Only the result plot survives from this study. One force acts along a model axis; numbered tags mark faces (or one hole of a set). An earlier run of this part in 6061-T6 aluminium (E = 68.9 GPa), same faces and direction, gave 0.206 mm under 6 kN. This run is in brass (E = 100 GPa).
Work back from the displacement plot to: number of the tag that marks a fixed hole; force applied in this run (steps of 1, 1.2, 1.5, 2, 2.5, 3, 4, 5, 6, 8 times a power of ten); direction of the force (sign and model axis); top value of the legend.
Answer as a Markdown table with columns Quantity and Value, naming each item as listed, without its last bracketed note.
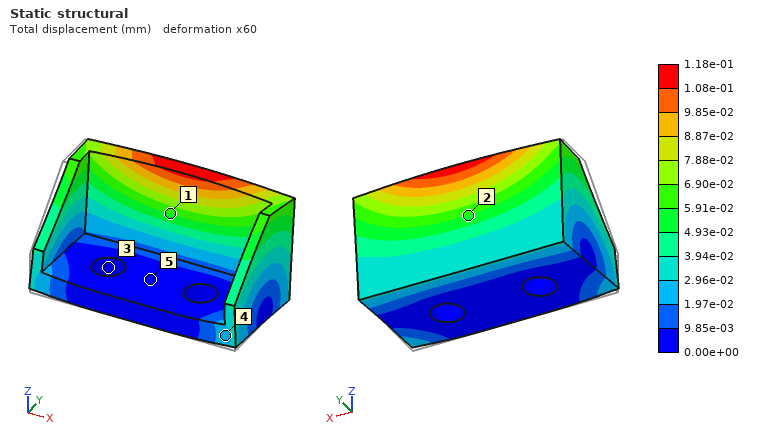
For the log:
| Quantity | Value |
|---|---|
| number of the tag that marks a fixed hole | 3 |
| force applied in this run | 5 kN |
| direction of the force | +Y |
| top value of the legend | 1.18e-01 mm |
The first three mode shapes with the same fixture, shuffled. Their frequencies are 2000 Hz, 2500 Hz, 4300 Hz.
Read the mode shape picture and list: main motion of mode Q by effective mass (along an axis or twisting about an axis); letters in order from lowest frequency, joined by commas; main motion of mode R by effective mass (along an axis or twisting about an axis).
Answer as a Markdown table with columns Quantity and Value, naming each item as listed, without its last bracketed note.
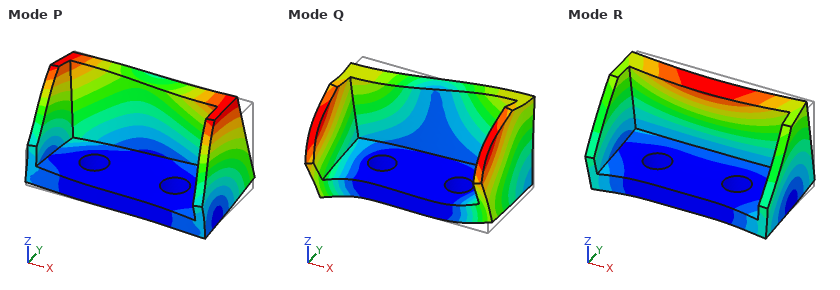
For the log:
| Quantity | Value |
|---|---|
| main motion of mode Q by effective mass | along X |
| letters in order from lowest frequency, joined by commas | R, P, Q |
| main motion of mode R by effective mass | along Y |
